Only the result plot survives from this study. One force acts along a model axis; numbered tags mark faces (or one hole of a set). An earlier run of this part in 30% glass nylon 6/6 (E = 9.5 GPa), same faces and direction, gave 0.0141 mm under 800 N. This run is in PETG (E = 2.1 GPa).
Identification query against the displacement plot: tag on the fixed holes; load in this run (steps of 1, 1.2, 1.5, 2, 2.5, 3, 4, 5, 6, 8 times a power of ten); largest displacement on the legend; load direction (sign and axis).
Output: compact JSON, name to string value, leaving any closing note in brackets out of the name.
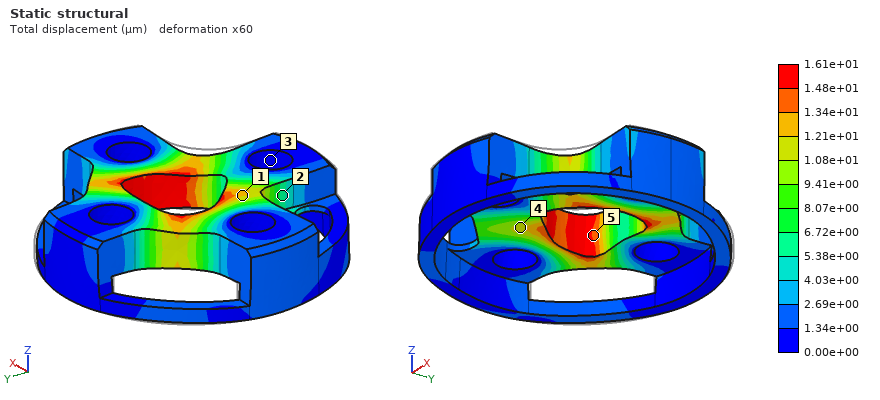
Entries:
{"tag on the fixed holes": "3", "load in this run": "200 N", "largest displacement on the legend": "1.61e+01 µm", "load direction": "+Y"}
